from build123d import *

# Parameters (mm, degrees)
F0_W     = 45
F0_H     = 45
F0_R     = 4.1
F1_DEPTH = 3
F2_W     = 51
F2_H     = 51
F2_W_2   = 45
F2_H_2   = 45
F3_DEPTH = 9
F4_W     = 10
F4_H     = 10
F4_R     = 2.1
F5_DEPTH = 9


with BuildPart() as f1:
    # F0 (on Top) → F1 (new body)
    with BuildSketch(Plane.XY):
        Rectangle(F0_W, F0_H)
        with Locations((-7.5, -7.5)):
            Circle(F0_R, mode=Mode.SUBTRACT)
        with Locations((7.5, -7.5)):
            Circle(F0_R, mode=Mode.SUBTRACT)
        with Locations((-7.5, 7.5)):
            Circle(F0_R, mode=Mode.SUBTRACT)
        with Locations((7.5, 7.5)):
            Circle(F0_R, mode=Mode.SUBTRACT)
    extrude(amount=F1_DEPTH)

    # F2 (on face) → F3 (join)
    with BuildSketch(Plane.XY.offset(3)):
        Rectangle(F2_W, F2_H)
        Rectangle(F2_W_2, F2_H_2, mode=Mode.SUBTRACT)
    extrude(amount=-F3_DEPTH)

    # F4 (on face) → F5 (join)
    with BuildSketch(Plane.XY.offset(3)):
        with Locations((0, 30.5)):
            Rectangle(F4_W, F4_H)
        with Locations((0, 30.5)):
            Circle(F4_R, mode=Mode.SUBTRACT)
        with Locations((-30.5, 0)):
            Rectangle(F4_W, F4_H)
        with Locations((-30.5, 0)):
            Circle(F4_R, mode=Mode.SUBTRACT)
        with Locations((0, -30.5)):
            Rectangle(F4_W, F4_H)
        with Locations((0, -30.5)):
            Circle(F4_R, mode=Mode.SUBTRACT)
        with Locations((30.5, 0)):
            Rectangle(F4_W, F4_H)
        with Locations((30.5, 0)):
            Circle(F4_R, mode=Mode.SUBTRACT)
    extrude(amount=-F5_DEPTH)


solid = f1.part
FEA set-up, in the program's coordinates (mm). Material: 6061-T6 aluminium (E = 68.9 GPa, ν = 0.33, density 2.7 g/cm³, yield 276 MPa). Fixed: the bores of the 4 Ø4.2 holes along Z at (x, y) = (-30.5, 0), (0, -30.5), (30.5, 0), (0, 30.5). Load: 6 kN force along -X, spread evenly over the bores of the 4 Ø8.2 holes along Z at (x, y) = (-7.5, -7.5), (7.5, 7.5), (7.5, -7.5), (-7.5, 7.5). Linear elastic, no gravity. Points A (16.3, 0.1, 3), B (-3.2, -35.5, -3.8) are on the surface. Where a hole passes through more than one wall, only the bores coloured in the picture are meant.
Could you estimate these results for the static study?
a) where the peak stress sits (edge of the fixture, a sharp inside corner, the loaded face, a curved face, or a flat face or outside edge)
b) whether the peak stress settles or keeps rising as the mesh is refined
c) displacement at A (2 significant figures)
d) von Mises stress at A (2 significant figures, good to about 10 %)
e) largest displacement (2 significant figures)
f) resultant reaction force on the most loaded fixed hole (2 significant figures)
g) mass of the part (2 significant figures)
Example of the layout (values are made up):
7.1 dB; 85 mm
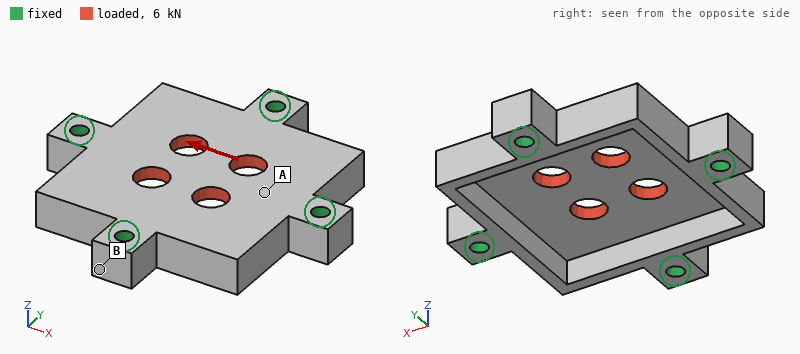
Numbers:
edge of the fixture; keeps rising; 11 µm; 50 MPa; 19 µm; 2.0 kN; 37 g
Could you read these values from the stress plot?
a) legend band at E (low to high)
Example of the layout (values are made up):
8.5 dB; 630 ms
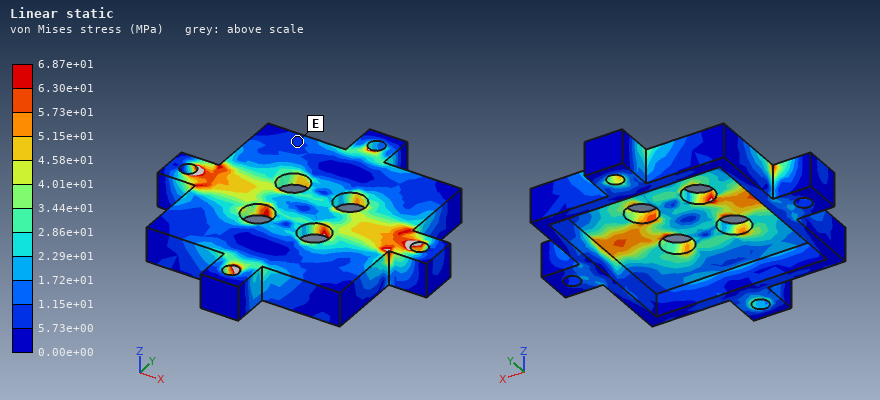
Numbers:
5.73e+00 to 1.15e+01 MPa
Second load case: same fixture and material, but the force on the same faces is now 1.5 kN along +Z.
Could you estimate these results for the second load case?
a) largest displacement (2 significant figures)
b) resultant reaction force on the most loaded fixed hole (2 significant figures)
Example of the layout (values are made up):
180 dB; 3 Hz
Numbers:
92 µm; 510 N
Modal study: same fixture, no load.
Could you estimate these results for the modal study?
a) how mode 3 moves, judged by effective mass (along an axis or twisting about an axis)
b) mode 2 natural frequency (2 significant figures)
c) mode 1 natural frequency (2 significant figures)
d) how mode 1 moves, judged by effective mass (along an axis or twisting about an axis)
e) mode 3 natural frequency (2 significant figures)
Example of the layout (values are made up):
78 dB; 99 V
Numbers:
twisting about Y; 12 kHz; 10 kHz; along Z; 13 kHz
